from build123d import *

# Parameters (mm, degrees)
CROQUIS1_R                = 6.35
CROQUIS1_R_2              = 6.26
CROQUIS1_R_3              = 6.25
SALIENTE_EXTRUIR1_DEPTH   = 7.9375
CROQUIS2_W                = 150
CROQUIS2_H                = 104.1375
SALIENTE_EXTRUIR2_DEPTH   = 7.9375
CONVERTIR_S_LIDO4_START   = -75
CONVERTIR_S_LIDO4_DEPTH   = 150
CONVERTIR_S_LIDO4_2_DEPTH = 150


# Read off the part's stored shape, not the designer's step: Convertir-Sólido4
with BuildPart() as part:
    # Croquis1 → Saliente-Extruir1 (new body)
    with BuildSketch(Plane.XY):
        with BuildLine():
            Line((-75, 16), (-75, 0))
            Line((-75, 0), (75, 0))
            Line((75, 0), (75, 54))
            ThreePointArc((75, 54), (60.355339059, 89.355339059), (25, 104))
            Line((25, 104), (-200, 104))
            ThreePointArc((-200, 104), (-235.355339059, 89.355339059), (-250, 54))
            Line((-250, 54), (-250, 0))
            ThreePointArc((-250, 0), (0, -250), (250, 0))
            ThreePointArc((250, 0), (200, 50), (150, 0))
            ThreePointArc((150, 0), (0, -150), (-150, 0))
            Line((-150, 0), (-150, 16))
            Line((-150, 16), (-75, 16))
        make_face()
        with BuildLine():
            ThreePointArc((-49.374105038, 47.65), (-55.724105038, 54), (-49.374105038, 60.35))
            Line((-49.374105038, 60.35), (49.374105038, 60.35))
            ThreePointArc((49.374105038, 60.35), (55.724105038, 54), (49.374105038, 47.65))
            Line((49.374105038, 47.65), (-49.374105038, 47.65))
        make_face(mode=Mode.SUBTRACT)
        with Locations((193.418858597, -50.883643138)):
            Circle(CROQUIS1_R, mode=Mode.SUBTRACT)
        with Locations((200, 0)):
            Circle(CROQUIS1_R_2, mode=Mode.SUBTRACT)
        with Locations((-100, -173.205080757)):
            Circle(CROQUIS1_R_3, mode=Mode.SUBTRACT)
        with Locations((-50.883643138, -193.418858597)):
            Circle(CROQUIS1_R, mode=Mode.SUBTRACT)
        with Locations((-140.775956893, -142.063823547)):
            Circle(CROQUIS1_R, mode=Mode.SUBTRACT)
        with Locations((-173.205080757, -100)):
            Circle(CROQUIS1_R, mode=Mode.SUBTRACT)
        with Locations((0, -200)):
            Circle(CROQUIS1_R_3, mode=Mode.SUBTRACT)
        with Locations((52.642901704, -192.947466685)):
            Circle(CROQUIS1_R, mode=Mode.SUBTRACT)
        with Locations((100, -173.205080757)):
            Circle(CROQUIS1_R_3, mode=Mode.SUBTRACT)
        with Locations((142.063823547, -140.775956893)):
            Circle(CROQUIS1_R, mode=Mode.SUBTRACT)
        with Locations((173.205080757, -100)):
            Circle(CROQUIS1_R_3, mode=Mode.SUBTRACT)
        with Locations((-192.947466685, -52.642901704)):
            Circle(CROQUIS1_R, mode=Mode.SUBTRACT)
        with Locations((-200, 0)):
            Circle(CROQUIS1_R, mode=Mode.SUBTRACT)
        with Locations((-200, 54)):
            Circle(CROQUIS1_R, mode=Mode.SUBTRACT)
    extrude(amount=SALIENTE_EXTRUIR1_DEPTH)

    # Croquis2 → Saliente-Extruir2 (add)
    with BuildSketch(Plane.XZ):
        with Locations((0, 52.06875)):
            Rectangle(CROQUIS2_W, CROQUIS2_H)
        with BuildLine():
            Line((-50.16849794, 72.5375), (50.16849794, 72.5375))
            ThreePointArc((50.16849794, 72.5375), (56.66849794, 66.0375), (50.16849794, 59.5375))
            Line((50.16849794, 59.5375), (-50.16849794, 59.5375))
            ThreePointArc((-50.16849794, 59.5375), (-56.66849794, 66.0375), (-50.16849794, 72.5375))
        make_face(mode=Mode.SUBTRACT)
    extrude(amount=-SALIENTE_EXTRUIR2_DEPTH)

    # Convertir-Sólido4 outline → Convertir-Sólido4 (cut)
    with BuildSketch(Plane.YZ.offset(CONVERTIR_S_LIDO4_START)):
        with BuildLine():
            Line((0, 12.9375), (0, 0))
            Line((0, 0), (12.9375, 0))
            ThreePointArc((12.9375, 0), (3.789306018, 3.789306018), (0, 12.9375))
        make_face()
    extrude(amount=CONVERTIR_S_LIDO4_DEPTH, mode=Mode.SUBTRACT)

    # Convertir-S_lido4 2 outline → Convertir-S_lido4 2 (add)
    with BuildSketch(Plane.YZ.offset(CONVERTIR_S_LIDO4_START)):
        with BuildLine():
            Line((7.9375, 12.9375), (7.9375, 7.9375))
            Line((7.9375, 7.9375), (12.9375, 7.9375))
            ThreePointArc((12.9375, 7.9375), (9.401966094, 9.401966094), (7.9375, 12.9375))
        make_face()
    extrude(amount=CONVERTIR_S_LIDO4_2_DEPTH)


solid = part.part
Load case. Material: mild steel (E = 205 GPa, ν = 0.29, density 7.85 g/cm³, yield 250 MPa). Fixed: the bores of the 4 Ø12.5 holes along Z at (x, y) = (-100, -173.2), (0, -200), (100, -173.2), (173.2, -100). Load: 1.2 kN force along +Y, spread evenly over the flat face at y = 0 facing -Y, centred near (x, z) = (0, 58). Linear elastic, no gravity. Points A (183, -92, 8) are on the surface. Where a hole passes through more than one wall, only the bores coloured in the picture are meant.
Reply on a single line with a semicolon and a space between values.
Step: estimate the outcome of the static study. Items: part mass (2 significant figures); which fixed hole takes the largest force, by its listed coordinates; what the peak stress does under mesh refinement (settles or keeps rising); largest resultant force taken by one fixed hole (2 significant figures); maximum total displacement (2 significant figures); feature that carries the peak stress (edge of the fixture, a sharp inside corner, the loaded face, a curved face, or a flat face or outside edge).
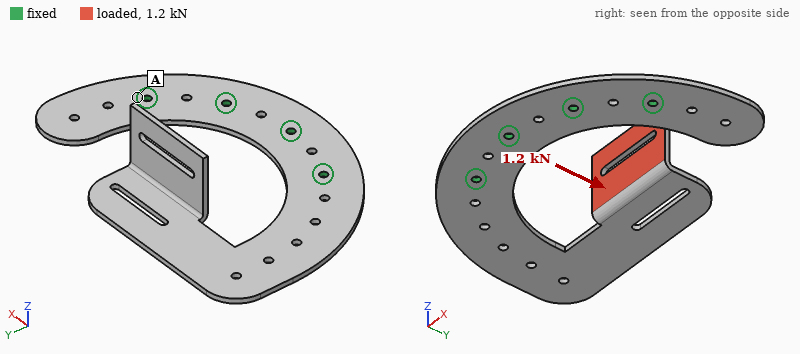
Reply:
6.7 kg; (0, -200); keeps rising; 880 N; 3.4 mm; a sharp inside corner
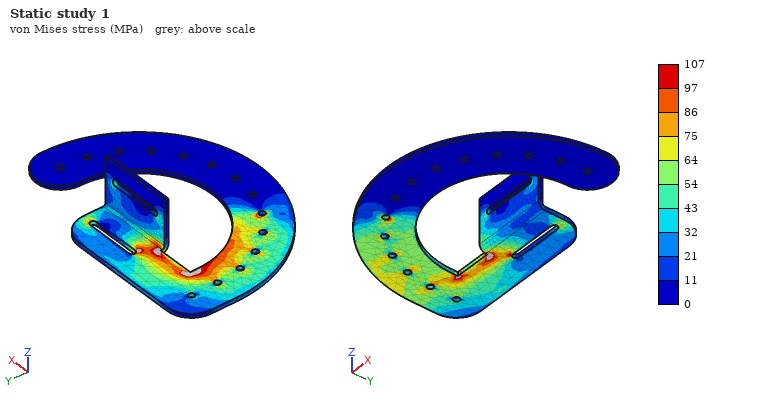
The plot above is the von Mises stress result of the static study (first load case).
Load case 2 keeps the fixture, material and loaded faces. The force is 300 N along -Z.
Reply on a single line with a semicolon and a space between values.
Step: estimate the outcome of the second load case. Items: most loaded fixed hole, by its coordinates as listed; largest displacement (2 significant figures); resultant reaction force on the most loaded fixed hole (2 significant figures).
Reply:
(-100, -173.2); 4.4 mm; 290 N
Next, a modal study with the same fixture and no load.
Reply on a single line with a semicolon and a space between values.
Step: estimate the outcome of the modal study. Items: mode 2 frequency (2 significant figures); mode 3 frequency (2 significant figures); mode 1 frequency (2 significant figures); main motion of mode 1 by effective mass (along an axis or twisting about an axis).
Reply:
61 Hz; 160 Hz; 35 Hz; along Z
